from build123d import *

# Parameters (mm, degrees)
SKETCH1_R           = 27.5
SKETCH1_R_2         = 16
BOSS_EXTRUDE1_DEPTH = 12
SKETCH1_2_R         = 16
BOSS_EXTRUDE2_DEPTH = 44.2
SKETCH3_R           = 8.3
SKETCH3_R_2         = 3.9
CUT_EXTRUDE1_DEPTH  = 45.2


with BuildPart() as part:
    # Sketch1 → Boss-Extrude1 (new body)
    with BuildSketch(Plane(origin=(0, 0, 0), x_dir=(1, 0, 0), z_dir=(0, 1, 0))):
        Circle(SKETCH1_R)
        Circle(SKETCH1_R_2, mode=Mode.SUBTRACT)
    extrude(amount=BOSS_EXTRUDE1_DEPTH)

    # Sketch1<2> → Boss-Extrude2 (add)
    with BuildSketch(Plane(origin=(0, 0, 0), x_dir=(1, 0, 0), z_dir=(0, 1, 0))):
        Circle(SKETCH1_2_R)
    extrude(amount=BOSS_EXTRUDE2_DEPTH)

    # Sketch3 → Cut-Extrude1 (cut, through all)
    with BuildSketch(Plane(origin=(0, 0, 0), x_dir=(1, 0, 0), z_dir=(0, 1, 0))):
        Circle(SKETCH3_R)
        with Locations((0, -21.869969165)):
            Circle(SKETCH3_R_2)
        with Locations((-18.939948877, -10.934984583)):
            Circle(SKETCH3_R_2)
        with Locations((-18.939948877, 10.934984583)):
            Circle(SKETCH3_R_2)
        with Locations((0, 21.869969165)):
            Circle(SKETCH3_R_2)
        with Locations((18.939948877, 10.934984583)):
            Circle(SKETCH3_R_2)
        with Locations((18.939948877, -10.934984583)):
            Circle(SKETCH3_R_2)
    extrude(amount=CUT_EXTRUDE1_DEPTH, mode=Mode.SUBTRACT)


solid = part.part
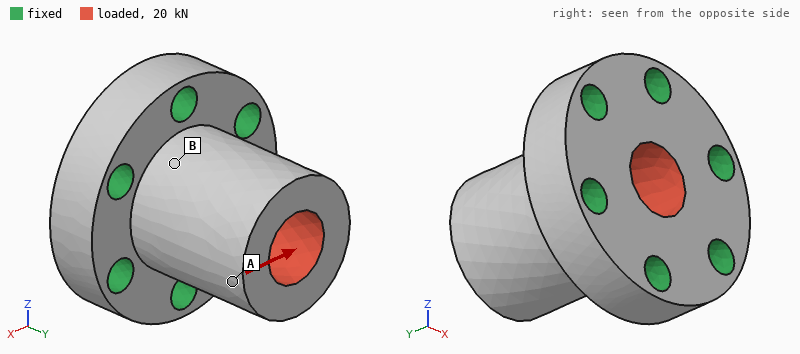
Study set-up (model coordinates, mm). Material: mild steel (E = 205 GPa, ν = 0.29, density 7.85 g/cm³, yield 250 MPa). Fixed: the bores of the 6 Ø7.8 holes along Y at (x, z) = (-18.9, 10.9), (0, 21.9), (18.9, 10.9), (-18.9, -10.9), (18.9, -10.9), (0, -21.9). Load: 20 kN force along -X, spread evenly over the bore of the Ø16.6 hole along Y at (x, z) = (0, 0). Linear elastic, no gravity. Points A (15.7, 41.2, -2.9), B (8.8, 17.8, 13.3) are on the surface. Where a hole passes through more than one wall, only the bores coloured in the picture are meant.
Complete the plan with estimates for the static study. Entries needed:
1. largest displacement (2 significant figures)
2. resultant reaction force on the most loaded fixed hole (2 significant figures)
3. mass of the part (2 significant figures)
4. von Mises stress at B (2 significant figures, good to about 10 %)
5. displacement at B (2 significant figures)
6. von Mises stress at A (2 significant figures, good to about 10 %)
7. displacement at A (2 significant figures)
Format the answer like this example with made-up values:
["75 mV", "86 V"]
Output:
["22 µm", "6.4 kN", "320 g", "44 MPa", "5.7 µm", "13 MPa", "21 µm"]
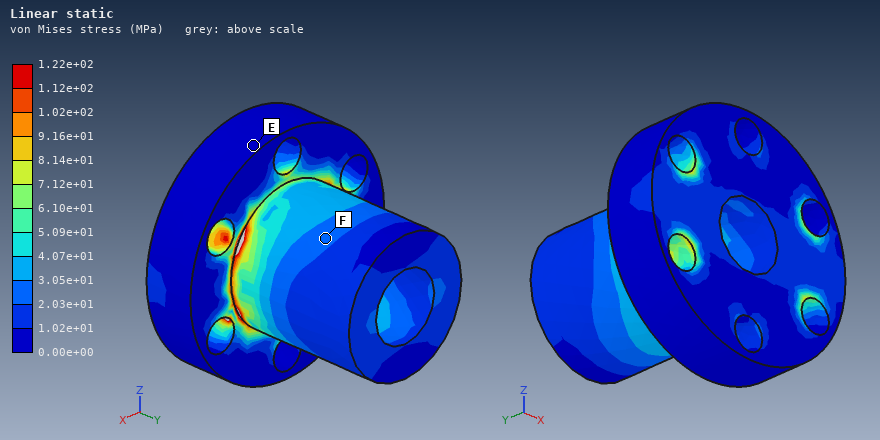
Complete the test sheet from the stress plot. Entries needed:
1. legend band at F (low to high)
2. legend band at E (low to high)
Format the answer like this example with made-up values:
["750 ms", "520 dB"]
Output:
["2.03e+01 to 3.05e+01 MPa", "0.00e+00 to 1.02e+01 MPa"]
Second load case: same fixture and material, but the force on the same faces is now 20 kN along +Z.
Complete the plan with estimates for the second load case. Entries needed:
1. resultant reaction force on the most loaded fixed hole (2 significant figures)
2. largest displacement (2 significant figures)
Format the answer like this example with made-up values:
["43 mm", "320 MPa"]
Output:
["7.3 kN", "22 µm"]
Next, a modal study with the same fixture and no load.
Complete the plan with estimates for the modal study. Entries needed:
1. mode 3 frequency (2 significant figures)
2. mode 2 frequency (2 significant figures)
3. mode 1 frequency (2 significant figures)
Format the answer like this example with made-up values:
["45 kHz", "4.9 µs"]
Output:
["22 kHz", "12 kHz", "12 kHz"]
